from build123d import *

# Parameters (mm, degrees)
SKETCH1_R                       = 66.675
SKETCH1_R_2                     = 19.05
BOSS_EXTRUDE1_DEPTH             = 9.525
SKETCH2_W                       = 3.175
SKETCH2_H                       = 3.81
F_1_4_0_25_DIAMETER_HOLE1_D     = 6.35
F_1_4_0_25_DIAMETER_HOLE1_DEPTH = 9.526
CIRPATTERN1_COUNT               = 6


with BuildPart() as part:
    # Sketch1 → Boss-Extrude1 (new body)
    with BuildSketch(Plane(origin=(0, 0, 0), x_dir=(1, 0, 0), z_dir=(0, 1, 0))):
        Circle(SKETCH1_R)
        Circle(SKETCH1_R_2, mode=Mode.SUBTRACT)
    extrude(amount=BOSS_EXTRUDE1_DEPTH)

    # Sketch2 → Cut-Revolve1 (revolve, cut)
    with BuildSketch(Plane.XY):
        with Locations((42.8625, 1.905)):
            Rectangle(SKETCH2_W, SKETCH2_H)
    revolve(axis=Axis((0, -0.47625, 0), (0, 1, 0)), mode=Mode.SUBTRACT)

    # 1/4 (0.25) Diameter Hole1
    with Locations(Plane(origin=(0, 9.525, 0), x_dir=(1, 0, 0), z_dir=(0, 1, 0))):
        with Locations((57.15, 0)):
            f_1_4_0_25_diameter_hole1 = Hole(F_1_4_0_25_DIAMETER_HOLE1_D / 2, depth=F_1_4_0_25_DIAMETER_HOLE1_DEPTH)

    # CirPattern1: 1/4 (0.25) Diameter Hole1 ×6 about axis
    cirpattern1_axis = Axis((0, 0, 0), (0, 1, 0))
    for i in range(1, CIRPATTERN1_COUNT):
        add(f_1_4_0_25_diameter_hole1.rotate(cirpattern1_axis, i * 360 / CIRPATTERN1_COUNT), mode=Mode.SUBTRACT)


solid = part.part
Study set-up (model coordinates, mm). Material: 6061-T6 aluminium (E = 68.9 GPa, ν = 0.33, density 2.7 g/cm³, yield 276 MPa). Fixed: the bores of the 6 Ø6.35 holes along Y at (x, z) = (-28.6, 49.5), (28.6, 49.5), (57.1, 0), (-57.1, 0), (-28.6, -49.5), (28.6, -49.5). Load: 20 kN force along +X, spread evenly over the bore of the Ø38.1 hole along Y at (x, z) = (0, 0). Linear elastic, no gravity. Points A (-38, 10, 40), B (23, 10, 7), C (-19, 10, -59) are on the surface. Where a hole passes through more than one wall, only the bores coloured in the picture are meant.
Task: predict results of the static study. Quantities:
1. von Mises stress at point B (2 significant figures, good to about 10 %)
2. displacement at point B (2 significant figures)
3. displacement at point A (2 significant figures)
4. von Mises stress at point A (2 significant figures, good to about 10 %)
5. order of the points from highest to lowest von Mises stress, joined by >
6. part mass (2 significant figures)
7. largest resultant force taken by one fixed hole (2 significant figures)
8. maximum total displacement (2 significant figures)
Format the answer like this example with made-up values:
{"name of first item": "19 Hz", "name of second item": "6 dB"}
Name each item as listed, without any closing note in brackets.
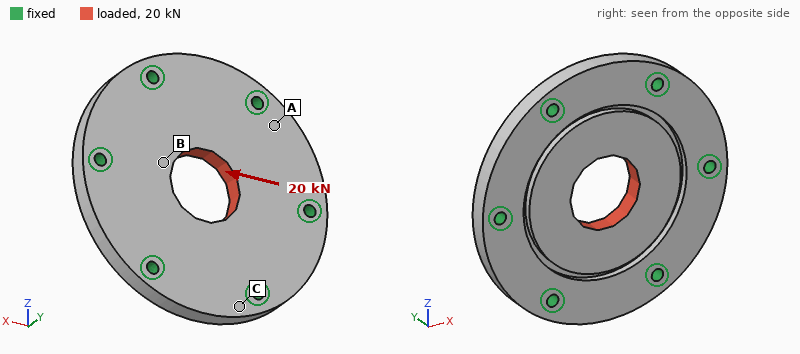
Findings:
{"von Mises stress at point B": "18 MPa", "displacement at point B": "11 µm", "displacement at point A": "4.8 µm", "von Mises stress at point A": "11 MPa", "order of the points from highest to lowest von Mises stress, joined by >": "B > A > C", "part mass": "320 g", "largest resultant force taken by one fixed hole": "4.7 kN", "maximum total displacement": "15 µm"}
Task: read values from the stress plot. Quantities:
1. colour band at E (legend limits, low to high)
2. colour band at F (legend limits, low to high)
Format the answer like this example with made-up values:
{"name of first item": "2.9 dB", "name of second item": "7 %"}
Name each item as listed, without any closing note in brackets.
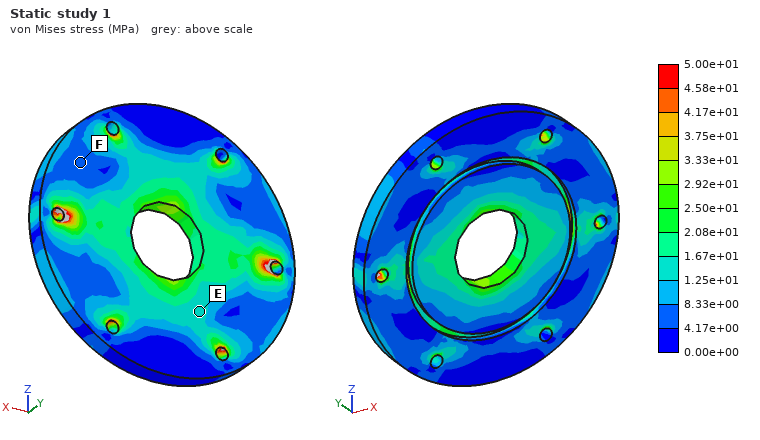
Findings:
{"colour band at E": "1.25e+01 to 1.67e+01 MPa", "colour band at F": "4.17e+00 to 8.33e+00 MPa"}
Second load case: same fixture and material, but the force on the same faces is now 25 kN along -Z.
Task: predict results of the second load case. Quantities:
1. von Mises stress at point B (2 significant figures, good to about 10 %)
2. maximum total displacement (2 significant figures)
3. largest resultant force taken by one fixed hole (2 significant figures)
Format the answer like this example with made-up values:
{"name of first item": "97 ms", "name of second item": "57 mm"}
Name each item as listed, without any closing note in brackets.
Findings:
{"von Mises stress at point B": "25 MPa", "maximum total displacement": "19 µm", "largest resultant force taken by one fixed hole": "5.2 kN"}
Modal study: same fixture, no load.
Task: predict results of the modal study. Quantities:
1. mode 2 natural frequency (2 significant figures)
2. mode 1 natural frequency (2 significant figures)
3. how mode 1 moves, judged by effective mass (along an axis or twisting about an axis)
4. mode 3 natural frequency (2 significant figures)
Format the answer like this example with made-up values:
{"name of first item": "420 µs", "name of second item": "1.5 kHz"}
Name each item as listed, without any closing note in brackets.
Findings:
{"mode 2 natural frequency": "9700 Hz", "mode 1 natural frequency": "6000 Hz", "how mode 1 moves, judged by effective mass": "along Y", "mode 3 natural frequency": "9700 Hz"}
